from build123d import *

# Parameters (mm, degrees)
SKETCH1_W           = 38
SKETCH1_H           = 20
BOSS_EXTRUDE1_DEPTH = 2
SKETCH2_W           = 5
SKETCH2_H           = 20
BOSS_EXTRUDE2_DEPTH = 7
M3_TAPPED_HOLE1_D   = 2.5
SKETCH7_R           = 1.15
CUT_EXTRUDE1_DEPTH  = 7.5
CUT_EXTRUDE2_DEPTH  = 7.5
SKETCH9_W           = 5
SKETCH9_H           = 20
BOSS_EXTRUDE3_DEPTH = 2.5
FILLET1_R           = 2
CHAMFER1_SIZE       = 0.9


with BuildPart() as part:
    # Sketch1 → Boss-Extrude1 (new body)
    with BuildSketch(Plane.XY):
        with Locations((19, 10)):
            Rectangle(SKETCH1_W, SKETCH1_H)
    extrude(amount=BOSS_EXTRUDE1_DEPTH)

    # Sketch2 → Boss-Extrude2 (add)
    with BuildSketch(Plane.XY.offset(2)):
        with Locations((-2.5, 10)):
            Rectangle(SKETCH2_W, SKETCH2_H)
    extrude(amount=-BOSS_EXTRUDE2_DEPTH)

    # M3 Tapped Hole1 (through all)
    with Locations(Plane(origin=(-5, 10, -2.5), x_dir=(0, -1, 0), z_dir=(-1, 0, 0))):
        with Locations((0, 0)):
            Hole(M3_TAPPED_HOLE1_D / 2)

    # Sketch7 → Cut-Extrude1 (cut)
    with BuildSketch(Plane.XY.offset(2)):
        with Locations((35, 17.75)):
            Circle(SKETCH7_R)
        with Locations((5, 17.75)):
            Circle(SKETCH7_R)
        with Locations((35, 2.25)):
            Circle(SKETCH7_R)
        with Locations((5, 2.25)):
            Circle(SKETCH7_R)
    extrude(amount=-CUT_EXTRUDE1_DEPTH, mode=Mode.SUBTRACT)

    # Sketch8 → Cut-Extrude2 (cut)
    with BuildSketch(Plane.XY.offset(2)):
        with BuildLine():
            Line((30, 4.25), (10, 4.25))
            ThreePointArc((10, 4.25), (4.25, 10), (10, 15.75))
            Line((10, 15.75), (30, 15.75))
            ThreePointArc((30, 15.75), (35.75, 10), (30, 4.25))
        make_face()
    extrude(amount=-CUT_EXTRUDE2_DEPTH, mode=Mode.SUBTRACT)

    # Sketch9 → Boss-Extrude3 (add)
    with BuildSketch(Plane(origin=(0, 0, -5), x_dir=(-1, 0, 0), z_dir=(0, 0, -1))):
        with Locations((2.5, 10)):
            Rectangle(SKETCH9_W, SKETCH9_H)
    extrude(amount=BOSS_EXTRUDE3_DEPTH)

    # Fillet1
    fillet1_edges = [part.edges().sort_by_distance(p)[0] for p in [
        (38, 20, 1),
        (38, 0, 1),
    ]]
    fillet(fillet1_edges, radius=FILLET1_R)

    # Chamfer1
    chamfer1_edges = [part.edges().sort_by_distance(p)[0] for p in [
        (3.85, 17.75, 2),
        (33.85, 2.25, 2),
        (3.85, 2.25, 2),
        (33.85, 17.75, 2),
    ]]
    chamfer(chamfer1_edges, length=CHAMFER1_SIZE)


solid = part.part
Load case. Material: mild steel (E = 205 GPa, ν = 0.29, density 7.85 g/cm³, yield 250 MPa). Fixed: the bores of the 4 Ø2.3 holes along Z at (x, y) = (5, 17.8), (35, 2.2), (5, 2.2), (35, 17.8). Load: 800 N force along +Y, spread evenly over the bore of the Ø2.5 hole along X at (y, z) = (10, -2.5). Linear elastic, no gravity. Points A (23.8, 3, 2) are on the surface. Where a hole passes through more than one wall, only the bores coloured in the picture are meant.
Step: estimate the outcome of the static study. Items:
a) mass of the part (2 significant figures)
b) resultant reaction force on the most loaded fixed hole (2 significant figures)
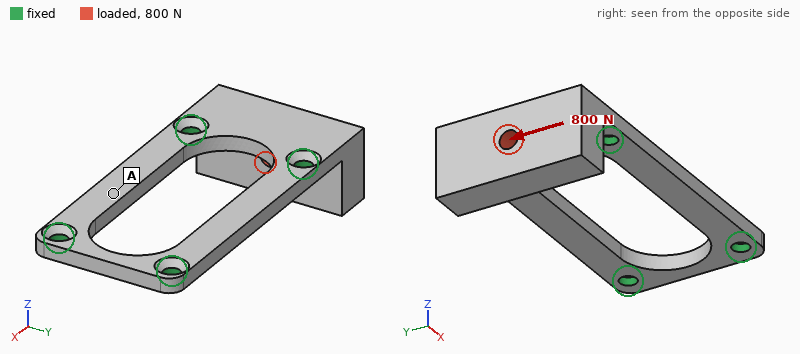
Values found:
14 g
550 N
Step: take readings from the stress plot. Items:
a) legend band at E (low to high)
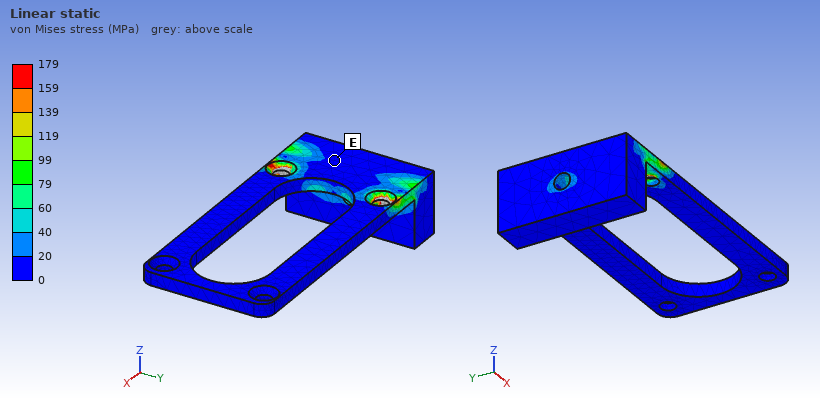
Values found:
0 to 20 MPa
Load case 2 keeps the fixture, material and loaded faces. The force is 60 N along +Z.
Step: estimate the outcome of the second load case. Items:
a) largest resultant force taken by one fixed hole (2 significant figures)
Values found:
31 N
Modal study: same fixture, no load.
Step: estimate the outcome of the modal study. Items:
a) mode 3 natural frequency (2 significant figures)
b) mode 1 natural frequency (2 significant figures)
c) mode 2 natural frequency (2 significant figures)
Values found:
11 kHz
4600 Hz
11 kHz
